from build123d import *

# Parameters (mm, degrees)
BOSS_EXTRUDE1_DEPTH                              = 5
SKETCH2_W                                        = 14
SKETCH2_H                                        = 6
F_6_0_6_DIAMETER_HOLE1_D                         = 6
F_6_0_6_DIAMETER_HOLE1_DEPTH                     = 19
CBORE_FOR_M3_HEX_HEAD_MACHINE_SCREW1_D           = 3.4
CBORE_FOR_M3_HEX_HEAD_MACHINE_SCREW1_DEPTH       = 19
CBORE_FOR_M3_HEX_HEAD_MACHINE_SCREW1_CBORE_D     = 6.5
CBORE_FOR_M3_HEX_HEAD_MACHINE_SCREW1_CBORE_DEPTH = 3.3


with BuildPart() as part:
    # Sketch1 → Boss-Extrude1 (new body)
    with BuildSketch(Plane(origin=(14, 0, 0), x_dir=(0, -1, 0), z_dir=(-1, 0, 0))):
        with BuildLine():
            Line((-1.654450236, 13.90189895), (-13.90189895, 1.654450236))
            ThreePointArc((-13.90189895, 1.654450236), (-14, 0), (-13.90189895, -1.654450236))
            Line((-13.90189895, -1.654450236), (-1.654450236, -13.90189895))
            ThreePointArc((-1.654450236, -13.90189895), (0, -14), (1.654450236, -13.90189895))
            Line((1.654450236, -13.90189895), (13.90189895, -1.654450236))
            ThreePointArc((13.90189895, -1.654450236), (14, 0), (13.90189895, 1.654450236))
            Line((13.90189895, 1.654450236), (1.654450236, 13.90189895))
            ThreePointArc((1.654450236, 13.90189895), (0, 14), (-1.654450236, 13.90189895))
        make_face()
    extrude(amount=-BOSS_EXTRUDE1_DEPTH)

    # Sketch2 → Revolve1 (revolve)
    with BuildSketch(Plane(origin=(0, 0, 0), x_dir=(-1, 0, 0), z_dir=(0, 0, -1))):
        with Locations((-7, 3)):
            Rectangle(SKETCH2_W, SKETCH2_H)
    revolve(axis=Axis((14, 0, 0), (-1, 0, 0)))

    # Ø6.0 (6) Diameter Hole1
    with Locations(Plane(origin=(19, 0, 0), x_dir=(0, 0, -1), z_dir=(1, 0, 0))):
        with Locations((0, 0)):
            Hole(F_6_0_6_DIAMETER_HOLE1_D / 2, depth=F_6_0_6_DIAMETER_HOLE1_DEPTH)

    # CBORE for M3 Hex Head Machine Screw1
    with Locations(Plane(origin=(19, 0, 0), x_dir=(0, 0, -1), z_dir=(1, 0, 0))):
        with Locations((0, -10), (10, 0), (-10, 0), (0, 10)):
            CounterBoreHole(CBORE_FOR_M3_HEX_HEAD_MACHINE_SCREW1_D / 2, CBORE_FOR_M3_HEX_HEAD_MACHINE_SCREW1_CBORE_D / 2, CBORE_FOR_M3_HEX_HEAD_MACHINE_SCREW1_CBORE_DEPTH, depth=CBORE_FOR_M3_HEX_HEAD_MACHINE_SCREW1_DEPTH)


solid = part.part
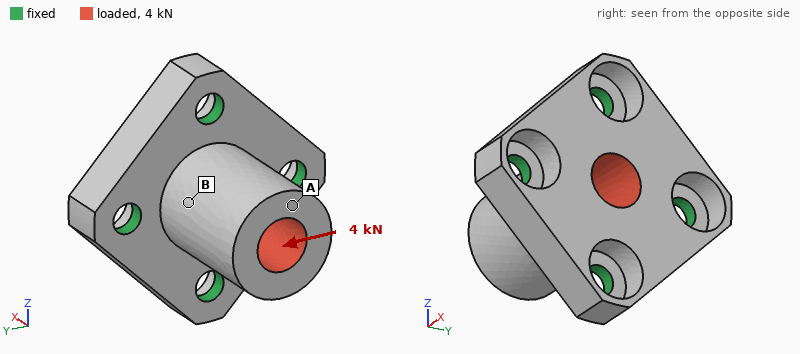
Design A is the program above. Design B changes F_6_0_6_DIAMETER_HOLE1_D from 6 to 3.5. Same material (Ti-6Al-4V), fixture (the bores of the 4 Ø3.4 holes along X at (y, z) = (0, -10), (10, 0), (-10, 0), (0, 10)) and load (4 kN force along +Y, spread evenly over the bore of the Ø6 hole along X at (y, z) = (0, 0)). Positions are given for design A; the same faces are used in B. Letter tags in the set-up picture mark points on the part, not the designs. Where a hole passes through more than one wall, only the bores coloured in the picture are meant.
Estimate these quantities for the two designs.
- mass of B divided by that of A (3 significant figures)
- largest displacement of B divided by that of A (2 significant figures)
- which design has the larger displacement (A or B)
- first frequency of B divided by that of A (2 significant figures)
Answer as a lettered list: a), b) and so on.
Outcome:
a) 1.12
b) 0.87
c) A
d) 0.98
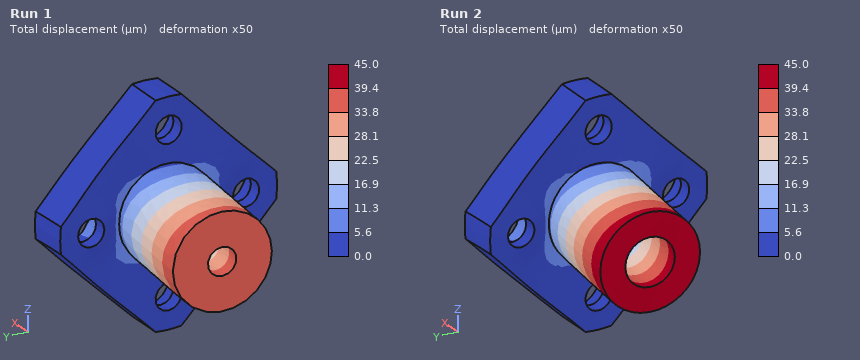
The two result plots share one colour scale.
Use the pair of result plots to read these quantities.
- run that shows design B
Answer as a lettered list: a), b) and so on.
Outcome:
a) Run 1
